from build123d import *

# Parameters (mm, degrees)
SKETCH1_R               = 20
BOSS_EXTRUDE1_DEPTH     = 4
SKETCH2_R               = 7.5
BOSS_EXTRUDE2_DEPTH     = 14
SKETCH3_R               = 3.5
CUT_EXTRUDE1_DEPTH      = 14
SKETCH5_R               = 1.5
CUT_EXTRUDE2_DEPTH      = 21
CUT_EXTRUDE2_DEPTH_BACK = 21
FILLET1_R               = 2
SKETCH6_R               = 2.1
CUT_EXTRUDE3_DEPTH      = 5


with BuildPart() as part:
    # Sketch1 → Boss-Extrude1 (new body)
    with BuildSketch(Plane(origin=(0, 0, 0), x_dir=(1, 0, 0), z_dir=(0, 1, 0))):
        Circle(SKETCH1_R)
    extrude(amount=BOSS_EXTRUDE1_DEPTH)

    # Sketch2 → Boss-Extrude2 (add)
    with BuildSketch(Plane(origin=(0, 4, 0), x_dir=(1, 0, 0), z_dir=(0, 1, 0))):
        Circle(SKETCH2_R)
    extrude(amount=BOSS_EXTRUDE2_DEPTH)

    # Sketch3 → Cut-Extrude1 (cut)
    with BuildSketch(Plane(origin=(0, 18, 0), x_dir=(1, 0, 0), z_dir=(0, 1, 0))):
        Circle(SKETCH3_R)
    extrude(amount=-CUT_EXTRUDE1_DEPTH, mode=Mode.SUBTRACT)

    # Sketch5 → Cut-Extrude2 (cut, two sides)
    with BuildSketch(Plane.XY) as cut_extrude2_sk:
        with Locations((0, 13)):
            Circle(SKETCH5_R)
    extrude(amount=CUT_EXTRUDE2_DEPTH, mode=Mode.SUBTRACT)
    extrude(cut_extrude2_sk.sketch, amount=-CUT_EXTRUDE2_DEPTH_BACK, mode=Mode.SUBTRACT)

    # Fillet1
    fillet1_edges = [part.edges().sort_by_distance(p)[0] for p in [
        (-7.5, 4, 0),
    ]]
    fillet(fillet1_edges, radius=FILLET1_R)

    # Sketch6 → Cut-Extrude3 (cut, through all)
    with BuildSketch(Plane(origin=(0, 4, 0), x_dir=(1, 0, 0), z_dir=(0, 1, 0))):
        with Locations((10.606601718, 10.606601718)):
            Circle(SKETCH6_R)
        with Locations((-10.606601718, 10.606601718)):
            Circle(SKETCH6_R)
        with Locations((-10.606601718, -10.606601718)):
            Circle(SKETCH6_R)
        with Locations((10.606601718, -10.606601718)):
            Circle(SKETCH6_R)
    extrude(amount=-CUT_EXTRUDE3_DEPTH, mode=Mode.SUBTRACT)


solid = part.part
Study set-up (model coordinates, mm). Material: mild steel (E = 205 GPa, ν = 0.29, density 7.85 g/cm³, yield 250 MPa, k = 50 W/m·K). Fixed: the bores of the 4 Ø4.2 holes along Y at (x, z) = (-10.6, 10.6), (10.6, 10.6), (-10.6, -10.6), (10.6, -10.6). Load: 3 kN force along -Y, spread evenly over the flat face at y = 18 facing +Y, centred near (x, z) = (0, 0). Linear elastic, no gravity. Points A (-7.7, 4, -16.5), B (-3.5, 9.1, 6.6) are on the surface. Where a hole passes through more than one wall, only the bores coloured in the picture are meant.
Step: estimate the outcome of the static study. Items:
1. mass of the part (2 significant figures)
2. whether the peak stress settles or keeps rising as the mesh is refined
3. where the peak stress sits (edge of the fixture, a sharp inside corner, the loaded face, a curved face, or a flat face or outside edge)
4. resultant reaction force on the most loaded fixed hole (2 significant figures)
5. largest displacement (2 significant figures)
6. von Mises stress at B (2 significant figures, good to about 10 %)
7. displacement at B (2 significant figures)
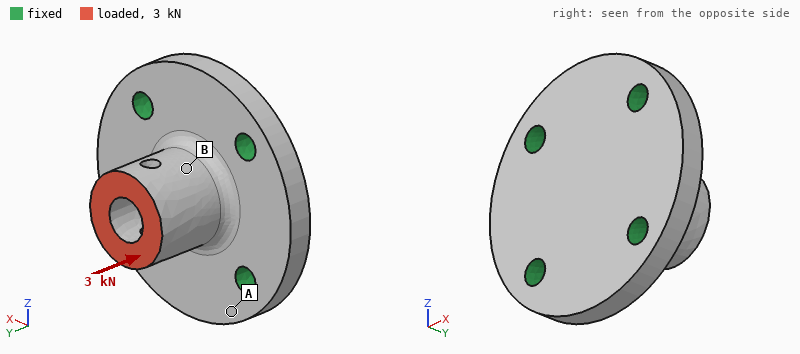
53 g
keeps rising
edge of the fixture
780 N
5.7 µm
25 MPa
4.4 µm
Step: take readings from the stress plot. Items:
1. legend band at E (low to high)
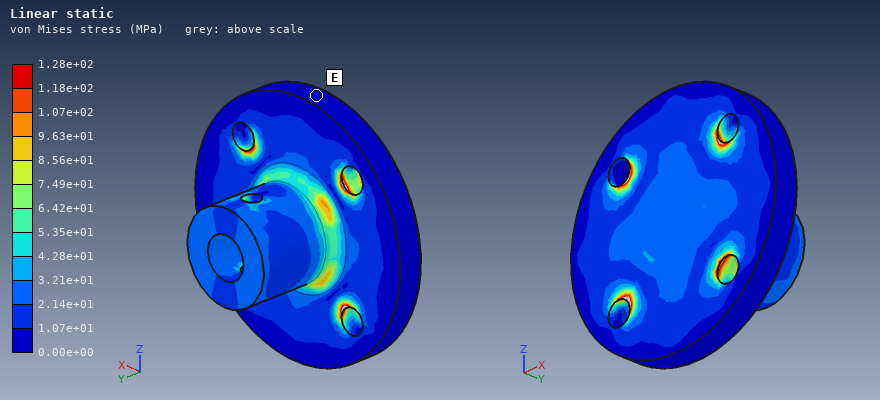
0.00e+00 to 1.07e+01 MPa
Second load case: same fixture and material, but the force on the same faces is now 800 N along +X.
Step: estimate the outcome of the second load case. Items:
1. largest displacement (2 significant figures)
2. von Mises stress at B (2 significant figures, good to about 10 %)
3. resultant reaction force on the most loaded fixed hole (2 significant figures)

7.9 µm
13 MPa
410 N
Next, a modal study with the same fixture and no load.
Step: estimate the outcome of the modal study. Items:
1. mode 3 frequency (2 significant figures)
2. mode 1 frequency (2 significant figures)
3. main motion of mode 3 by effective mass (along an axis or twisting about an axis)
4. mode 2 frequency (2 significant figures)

27 kHz
22 kHz
along Y
22 kHz
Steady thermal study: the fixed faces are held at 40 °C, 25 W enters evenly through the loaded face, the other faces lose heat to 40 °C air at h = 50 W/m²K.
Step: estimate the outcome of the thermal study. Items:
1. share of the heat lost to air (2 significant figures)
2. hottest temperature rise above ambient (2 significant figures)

12 %
70 K
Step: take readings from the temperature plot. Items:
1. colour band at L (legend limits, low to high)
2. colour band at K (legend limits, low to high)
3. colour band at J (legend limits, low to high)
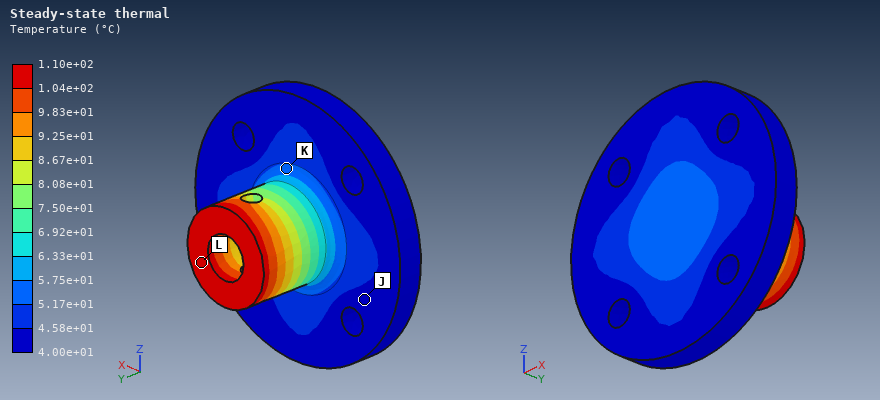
1.04e+02 to 1.10e+02 °C
5.17e+01 to 5.75e+01 °C
4.00e+01 to 4.58e+01 °C
